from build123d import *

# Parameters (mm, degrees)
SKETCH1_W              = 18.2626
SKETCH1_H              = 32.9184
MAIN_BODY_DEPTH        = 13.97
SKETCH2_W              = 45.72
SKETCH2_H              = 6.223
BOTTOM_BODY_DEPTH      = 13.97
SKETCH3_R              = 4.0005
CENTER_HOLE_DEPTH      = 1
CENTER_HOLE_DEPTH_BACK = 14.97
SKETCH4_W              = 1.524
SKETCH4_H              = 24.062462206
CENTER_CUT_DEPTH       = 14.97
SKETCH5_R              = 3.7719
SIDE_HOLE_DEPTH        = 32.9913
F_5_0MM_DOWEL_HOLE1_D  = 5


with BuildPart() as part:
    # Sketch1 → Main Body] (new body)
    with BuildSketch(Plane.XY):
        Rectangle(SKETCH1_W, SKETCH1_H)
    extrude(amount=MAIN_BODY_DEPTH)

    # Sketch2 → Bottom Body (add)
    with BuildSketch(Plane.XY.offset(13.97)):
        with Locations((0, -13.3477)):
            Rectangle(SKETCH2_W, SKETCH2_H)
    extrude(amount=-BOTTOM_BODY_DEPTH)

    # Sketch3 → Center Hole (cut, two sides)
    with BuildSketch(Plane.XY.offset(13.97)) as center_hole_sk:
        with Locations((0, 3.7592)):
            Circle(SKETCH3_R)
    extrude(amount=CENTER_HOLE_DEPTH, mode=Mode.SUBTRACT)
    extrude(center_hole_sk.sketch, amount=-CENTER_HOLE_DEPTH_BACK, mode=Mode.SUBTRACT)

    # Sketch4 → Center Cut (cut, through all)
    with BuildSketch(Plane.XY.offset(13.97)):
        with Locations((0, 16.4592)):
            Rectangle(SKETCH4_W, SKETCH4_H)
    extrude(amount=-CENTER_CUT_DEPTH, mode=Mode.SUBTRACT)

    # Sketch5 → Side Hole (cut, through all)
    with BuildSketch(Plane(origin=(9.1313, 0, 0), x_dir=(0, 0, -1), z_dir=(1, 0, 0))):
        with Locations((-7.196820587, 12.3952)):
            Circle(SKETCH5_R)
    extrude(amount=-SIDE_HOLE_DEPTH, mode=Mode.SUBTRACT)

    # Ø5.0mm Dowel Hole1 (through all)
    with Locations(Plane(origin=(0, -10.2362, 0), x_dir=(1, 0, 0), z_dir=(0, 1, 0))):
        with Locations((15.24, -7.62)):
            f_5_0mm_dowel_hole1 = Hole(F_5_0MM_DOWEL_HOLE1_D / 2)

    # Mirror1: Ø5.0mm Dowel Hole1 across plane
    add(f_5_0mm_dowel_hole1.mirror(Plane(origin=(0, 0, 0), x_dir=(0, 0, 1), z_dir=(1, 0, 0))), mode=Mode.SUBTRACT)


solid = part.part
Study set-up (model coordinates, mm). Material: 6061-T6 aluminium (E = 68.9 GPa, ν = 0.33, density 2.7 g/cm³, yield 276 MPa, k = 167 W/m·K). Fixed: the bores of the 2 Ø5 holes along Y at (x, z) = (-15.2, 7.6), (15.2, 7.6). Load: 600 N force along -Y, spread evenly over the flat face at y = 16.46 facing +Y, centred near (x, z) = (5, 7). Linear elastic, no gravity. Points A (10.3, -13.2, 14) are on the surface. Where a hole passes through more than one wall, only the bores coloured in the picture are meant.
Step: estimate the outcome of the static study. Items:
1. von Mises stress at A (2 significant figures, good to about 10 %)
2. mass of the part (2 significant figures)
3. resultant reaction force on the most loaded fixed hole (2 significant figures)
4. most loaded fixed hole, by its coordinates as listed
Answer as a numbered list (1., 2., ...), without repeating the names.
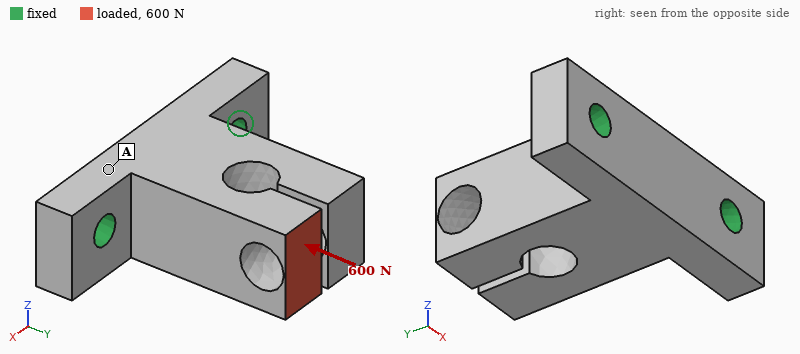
1. 9.3 MPa
2. 24 g
3. 440 N
4. (15.2, 7.6)
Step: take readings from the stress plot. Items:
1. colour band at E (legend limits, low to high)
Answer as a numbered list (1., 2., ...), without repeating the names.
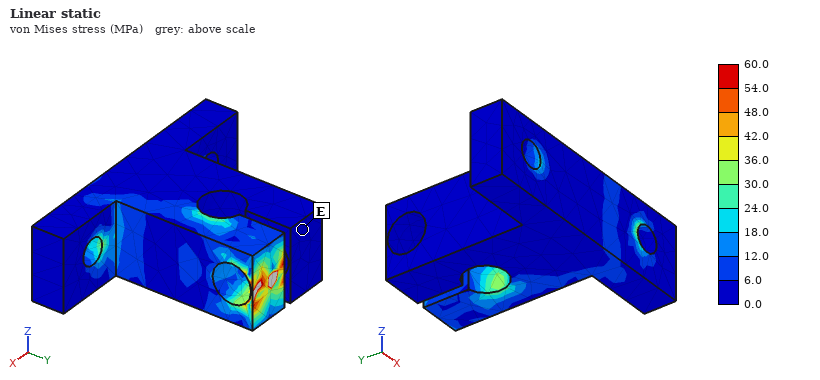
1. 0.0 to 6.0 MPa
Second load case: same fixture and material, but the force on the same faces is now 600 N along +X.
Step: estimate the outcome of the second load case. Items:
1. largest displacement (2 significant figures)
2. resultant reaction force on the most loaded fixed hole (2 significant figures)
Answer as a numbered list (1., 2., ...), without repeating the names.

1. 0.13 mm
2. 870 N
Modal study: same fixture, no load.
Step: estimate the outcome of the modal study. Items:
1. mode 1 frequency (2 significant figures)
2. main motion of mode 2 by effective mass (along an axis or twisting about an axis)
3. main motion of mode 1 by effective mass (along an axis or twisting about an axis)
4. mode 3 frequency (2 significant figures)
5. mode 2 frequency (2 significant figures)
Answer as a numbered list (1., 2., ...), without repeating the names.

1. 6000 Hz
2. along X
3. along Z
4. 12 kHz
5. 10000 Hz
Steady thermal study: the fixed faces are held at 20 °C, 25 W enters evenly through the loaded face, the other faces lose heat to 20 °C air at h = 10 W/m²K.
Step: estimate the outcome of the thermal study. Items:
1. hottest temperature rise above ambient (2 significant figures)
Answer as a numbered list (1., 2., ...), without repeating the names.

1. 64 K
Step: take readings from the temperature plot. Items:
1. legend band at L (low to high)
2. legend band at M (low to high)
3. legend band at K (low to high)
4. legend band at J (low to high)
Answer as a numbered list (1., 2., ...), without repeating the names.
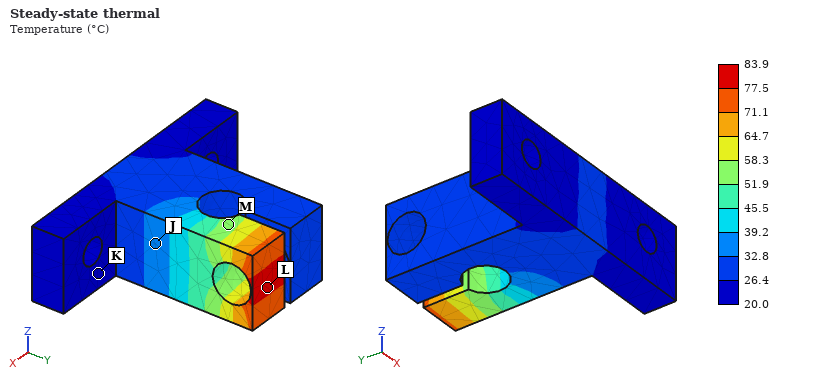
1. 77.5 to 83.9 °C
2. 51.9 to 58.3 °C
3. 20.0 to 26.4 °C
4. 32.8 to 39.2 °C
